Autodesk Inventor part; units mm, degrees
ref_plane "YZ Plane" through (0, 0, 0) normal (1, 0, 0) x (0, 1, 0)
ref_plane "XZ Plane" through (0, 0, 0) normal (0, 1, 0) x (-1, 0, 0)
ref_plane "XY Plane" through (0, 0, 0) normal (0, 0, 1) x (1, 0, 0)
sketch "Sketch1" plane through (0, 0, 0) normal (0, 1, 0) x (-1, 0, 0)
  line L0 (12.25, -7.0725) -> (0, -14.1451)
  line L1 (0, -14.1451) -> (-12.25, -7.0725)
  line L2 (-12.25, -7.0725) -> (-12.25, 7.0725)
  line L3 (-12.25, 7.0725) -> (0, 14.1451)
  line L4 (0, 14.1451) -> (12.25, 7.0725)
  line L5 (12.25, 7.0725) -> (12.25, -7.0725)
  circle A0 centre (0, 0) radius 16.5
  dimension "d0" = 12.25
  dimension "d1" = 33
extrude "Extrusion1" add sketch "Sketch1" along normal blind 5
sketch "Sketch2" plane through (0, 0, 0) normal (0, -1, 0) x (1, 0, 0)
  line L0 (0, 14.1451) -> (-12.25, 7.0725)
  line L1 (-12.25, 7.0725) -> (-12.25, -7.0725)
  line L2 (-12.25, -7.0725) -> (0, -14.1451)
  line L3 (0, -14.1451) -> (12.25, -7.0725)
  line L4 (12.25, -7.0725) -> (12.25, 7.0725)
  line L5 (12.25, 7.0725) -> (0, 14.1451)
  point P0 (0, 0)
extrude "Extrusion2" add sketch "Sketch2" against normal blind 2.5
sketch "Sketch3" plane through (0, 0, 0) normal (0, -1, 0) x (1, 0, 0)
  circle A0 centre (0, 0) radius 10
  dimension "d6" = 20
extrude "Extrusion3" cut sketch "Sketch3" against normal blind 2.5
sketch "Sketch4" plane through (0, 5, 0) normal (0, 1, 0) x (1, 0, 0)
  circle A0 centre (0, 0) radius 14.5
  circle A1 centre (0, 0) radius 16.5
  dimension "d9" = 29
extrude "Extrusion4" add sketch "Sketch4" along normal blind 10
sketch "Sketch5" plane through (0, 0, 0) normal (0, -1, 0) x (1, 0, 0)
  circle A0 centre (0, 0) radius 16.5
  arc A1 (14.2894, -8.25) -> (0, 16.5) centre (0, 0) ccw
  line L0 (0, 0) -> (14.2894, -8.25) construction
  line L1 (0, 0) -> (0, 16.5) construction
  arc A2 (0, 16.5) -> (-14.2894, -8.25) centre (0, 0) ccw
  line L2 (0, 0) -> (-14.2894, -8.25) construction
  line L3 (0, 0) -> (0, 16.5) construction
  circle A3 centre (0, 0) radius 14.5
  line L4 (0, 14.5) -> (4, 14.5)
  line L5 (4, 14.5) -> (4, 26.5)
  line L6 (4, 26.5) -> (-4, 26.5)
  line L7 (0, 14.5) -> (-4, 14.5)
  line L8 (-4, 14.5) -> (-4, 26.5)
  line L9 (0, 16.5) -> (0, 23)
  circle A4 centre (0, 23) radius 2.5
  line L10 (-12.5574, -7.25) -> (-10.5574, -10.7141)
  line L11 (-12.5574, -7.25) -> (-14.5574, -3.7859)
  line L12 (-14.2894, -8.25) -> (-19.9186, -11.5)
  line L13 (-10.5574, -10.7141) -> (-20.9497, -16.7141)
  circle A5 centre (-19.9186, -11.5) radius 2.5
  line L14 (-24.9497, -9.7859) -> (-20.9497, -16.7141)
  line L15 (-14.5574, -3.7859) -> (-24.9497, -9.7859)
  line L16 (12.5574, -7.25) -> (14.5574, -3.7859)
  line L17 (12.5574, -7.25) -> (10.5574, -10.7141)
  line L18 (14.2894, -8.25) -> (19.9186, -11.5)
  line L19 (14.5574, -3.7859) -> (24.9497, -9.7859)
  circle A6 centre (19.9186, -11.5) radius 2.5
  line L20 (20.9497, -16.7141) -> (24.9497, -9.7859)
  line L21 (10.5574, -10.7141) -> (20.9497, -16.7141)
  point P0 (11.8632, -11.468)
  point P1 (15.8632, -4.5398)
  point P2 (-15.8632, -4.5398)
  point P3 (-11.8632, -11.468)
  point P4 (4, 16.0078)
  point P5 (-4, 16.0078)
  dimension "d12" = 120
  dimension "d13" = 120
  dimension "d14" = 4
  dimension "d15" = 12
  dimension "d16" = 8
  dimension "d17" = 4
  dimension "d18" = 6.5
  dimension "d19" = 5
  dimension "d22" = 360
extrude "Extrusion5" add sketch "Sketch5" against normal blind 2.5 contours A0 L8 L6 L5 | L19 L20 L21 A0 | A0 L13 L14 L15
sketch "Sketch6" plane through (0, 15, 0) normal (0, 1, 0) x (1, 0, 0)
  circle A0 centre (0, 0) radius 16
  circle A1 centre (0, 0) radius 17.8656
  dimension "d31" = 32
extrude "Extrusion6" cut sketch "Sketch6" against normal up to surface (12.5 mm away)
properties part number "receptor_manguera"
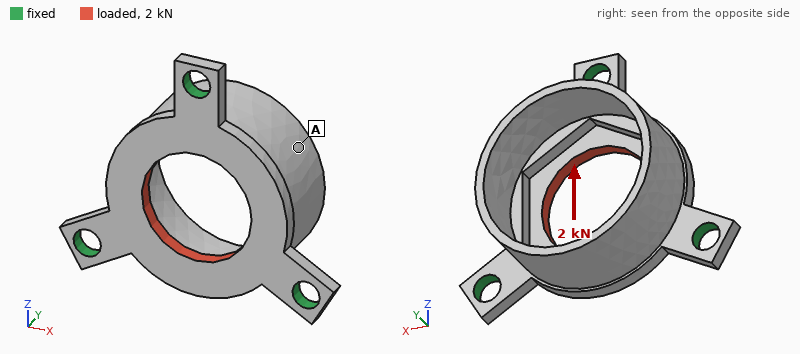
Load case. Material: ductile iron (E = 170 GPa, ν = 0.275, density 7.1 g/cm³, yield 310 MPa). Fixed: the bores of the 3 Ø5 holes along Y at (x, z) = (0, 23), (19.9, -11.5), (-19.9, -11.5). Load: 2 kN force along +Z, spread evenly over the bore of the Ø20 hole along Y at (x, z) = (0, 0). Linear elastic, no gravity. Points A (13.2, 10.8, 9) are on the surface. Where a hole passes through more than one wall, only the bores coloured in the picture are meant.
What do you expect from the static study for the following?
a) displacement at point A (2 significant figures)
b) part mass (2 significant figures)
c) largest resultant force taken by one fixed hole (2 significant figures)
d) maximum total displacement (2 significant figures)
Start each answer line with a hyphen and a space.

- 5.9 µm
- 28 g
- 690 N
- 13 µm
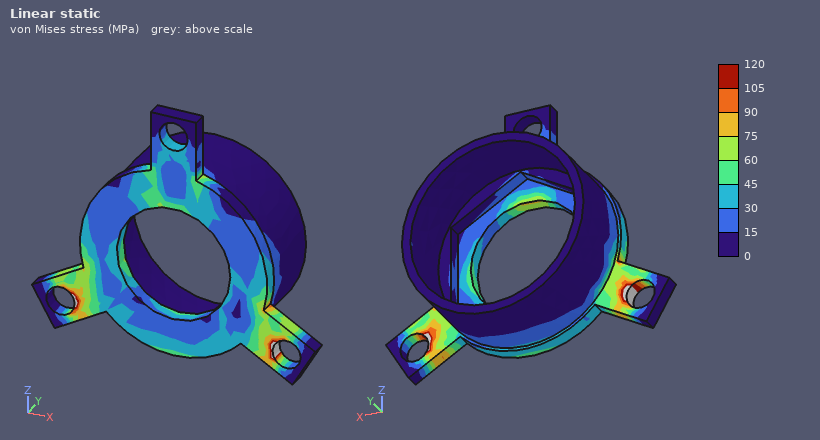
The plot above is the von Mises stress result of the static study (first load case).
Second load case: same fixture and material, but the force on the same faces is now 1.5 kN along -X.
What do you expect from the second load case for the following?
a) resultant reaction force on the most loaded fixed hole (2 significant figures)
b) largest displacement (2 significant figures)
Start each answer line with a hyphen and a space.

- 530 N
- 8.6 µm
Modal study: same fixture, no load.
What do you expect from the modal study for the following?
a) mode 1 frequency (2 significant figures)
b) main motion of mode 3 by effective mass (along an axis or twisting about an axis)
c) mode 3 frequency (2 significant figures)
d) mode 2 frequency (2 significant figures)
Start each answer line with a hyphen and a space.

- 7200 Hz
- along Y
- 10 kHz
- 7200 Hz
